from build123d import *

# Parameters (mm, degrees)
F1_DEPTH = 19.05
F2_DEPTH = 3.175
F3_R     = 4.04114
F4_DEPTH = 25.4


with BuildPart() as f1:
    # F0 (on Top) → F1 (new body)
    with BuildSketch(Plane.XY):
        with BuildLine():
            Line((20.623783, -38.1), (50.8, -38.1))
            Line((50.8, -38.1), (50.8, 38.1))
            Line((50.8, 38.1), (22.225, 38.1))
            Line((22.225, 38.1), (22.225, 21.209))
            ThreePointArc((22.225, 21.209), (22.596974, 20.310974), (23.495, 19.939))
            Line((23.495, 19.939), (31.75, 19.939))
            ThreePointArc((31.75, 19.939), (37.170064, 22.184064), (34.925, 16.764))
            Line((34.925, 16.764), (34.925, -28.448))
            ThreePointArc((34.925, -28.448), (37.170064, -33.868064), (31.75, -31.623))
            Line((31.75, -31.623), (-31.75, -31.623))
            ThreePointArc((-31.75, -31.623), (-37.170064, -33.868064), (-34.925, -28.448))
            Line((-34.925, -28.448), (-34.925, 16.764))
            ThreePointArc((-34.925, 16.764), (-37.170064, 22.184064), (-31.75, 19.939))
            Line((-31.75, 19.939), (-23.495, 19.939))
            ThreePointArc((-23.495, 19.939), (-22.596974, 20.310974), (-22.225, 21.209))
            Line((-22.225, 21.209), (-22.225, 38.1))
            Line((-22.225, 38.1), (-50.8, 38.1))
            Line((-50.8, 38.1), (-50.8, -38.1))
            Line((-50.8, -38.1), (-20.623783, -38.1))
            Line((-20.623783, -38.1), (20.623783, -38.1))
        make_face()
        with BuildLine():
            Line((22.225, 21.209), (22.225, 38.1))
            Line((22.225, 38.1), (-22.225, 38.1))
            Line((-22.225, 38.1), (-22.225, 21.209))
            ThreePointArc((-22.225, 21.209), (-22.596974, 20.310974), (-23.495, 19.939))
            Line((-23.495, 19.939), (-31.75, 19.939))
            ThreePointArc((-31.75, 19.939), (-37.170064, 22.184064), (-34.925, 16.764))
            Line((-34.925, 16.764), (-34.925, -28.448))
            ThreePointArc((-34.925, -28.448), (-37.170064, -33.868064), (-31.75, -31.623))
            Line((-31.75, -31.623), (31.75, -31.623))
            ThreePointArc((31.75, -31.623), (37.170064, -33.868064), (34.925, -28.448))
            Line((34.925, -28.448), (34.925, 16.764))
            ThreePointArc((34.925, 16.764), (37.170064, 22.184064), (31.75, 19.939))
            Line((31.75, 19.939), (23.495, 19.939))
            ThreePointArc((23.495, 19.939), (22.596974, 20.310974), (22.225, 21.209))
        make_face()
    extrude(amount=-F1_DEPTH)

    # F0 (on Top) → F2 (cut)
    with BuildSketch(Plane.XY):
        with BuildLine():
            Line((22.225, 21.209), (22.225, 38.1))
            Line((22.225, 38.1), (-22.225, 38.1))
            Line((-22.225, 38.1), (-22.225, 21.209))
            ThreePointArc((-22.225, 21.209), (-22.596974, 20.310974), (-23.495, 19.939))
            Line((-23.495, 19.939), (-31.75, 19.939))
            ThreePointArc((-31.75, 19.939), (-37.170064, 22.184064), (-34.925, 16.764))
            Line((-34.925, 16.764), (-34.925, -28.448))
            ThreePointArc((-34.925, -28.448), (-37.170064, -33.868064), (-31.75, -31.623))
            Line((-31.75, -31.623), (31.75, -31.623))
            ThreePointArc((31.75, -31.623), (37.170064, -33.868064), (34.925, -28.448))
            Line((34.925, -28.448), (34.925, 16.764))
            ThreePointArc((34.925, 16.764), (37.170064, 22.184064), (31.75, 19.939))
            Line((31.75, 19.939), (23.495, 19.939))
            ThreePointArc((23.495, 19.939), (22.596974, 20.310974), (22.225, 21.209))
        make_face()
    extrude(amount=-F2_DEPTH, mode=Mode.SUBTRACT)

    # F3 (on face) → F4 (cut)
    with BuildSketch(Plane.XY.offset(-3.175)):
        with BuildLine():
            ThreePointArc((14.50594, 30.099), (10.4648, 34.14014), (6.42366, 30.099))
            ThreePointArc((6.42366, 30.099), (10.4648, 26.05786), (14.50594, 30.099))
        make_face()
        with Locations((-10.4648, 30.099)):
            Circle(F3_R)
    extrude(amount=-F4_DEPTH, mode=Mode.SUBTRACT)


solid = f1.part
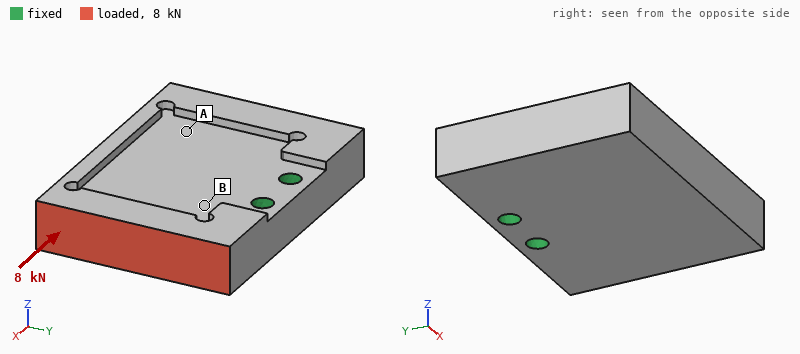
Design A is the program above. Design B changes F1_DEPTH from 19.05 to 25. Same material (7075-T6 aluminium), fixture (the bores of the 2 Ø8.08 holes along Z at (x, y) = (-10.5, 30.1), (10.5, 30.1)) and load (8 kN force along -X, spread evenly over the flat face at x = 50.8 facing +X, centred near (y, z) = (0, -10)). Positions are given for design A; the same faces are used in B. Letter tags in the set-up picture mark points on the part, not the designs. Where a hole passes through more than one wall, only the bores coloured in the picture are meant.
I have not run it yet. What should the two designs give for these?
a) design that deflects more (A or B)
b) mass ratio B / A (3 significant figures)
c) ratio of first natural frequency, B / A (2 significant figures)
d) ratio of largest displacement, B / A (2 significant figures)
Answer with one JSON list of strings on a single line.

["A", "1.35", "1.3", "0.72"]
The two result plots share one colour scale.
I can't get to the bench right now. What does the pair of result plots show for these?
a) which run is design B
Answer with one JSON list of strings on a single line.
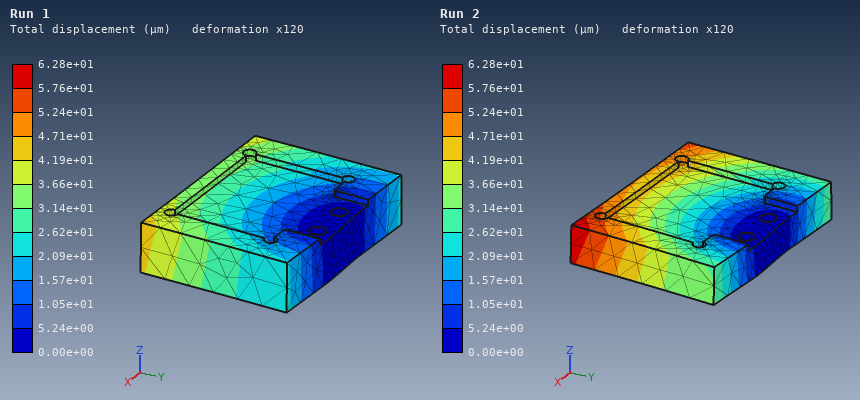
["Run 1"]
